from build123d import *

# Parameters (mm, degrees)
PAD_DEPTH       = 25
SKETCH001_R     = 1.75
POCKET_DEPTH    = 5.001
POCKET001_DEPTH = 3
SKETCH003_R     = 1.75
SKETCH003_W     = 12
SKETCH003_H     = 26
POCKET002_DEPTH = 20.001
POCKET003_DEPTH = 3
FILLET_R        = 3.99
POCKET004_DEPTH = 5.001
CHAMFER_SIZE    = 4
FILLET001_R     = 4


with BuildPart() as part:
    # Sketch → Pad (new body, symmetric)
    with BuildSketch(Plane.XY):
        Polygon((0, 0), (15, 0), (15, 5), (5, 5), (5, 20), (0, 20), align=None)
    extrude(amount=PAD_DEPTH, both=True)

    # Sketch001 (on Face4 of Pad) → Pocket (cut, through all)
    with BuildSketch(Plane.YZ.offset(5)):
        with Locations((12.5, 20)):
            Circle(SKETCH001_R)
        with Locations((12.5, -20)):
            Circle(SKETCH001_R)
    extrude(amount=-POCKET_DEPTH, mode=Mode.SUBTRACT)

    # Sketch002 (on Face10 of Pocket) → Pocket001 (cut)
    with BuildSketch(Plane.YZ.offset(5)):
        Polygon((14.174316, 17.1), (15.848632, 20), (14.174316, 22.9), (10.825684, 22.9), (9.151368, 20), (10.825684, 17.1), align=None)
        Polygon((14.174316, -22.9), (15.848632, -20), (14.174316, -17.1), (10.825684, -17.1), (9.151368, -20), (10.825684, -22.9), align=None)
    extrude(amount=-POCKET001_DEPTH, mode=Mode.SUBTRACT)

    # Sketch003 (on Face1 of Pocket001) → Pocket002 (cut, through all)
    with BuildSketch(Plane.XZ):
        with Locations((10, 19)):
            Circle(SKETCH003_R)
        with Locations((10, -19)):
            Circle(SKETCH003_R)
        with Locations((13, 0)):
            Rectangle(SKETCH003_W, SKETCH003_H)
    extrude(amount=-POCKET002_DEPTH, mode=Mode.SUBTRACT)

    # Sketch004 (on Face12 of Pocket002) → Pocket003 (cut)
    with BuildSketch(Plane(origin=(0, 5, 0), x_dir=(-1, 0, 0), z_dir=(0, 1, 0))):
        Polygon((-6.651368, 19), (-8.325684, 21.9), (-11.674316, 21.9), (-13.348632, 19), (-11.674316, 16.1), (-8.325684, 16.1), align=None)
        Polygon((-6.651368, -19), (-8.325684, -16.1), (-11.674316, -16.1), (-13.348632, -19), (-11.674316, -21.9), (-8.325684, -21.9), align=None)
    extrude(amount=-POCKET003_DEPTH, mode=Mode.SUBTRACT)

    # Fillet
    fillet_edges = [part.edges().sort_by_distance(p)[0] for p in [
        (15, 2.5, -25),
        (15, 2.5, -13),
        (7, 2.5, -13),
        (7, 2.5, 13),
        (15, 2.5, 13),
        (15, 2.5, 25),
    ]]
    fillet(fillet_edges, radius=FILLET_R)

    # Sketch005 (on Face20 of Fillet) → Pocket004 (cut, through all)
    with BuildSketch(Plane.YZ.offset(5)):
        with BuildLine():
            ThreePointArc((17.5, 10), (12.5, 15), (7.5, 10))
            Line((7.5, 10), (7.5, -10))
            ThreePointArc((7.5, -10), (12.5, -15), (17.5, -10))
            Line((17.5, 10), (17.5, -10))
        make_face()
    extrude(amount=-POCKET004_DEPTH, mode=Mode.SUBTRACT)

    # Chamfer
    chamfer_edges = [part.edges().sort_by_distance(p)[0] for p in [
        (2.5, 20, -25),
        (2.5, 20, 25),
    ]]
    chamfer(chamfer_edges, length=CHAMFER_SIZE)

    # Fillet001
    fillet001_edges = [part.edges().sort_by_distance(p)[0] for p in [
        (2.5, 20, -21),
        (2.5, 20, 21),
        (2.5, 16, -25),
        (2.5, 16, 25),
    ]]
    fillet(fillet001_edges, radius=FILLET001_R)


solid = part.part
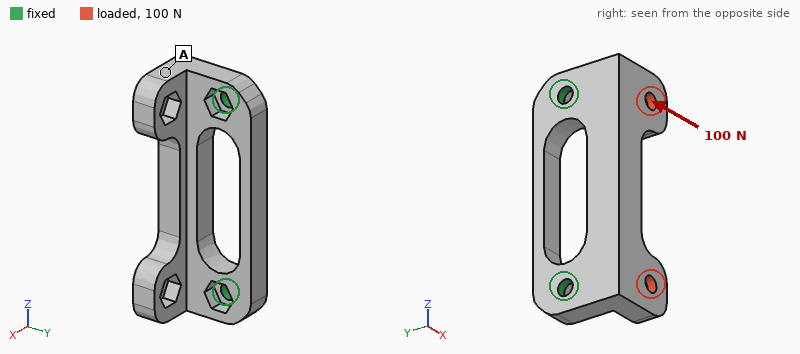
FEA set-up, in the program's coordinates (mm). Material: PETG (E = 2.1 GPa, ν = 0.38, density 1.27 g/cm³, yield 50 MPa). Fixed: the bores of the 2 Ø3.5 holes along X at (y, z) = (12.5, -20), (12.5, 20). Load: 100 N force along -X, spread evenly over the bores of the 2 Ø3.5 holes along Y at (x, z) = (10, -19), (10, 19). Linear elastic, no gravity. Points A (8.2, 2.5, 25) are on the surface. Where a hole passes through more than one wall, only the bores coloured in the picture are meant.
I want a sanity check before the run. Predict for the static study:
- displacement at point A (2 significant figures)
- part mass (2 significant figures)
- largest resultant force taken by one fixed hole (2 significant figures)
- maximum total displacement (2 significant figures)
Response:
0.34 mm
5.7 g
50 N
0.58 mm
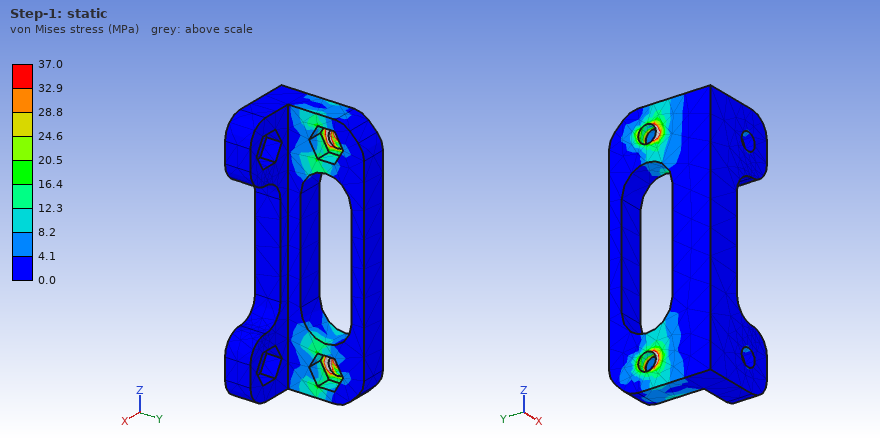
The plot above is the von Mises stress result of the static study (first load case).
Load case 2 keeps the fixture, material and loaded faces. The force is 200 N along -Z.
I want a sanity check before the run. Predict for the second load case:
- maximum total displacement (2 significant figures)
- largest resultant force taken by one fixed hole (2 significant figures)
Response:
0.23 mm
120 N
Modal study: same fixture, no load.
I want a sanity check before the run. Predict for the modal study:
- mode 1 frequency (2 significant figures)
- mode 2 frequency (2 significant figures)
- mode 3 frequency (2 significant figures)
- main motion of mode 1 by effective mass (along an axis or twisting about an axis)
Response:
1400 Hz
2400 Hz
3000 Hz
along X
